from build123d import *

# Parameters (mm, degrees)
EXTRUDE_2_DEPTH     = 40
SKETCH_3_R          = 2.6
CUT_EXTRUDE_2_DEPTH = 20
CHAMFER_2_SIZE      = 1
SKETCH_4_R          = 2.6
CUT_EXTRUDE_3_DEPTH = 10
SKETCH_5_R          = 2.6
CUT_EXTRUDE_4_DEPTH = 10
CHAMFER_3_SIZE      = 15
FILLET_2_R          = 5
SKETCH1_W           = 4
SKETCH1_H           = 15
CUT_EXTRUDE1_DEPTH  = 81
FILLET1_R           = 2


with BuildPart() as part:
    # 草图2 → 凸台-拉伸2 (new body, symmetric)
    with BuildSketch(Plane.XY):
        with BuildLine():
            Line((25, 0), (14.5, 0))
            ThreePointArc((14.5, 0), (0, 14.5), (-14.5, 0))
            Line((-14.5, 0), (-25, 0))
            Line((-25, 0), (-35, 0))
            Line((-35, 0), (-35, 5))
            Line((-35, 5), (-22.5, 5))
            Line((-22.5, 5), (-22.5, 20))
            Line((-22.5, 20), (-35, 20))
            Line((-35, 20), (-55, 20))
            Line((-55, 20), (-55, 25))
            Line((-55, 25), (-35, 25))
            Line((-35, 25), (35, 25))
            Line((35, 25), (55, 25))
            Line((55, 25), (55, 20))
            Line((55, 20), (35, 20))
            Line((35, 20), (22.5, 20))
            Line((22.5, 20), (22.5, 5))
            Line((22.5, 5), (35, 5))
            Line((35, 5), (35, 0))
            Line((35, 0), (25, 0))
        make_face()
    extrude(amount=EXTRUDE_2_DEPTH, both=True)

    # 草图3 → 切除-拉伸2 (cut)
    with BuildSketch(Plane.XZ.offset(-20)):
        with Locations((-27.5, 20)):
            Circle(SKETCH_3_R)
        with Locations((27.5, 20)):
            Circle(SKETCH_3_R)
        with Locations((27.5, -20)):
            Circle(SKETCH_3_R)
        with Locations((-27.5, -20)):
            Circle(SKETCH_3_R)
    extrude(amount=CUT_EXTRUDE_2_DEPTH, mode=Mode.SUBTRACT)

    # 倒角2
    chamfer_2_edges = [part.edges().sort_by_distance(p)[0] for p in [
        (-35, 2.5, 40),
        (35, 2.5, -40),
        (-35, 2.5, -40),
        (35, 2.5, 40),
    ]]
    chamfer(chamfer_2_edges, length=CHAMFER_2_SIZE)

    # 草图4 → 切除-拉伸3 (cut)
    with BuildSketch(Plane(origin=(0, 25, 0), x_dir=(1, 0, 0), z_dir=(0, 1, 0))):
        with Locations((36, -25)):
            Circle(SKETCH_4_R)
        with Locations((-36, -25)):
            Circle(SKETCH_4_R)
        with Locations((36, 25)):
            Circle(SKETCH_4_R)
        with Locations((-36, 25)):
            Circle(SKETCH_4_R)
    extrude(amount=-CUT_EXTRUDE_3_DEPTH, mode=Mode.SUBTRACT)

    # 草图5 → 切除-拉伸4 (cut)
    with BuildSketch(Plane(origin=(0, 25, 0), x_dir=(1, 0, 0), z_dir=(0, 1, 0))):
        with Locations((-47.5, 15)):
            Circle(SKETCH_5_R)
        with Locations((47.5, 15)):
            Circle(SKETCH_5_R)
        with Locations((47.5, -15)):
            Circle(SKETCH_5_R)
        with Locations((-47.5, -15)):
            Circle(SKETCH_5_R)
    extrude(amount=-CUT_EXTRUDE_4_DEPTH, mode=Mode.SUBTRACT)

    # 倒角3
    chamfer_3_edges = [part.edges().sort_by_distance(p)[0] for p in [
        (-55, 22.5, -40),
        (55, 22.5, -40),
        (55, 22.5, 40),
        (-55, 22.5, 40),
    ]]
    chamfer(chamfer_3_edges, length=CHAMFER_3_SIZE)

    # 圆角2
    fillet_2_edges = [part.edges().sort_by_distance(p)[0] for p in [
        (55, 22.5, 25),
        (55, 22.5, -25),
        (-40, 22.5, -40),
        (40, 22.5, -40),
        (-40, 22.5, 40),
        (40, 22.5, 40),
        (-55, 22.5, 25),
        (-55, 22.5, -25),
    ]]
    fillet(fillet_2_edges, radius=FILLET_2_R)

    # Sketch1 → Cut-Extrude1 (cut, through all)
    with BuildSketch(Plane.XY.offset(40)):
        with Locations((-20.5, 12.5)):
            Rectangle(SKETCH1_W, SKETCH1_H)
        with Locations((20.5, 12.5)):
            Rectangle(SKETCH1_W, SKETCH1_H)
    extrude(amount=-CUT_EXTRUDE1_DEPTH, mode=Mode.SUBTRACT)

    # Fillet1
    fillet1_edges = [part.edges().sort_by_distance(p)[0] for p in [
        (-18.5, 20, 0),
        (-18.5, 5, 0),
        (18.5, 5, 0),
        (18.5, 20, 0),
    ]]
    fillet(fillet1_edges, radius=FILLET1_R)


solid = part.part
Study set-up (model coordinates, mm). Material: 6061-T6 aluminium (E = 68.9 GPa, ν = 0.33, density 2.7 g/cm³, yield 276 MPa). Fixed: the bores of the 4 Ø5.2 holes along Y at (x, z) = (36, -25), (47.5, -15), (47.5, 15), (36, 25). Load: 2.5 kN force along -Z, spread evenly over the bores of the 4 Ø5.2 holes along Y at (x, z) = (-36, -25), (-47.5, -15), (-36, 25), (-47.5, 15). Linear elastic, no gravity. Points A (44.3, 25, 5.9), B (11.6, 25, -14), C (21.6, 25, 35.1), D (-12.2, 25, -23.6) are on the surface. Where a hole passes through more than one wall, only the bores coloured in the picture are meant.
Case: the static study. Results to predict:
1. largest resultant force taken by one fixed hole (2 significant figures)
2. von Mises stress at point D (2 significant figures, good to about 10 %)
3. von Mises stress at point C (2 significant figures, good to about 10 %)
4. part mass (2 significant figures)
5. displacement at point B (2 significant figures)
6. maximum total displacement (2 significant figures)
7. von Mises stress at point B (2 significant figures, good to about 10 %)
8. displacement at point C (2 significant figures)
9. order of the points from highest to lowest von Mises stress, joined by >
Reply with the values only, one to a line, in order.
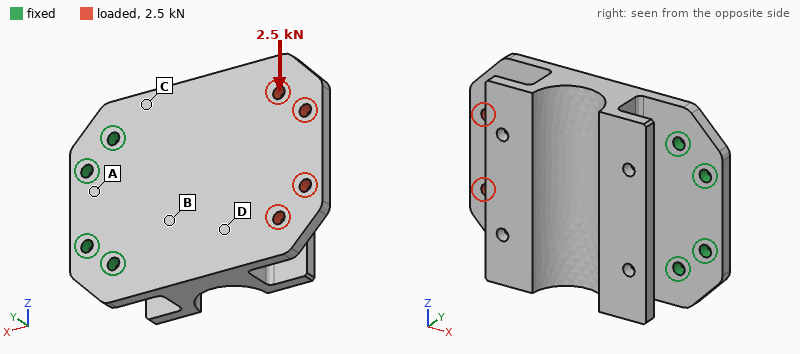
3.5 kN
11 MPa
15 MPa
230 g
16 µm
68 µm
21 MPa
16 µm
B > C > D > A
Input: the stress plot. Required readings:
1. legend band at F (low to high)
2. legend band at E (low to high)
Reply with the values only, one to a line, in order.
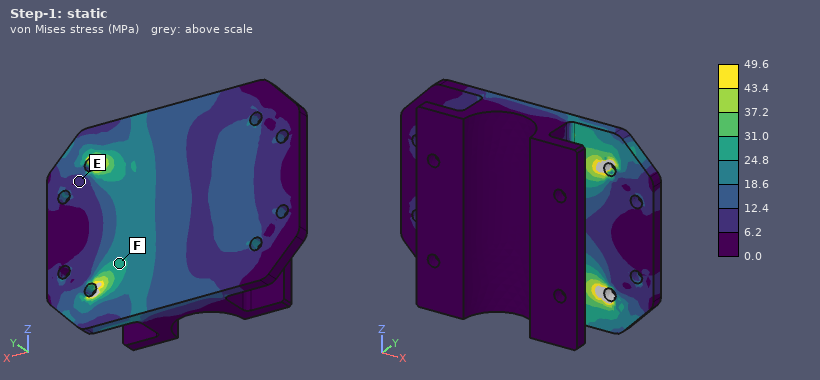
24.8 to 31.0 MPa
6.2 to 12.4 MPa
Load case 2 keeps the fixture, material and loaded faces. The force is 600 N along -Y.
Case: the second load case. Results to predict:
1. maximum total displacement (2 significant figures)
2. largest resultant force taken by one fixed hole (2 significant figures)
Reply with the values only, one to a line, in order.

1.3 mm
860 N
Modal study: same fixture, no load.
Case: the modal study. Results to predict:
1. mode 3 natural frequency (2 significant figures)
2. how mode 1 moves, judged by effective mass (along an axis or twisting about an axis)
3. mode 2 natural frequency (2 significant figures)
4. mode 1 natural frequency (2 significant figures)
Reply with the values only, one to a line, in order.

3400 Hz
along Y
2000 Hz
470 Hz
